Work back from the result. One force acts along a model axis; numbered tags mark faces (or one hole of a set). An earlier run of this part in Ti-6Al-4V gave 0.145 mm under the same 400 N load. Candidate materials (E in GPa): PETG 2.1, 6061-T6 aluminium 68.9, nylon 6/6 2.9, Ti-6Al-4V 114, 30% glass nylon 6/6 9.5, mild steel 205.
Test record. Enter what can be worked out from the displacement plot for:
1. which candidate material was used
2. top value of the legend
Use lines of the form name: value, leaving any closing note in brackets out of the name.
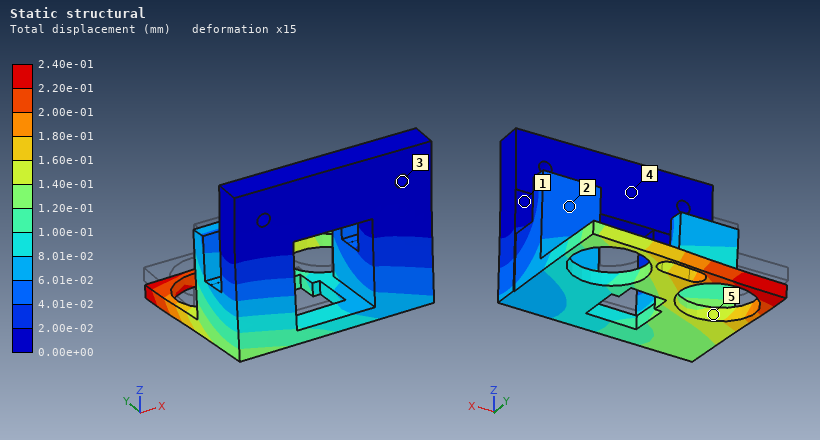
which candidate material was used: 6061-T6 aluminium
top value of the legend: 2.40e-01 mm
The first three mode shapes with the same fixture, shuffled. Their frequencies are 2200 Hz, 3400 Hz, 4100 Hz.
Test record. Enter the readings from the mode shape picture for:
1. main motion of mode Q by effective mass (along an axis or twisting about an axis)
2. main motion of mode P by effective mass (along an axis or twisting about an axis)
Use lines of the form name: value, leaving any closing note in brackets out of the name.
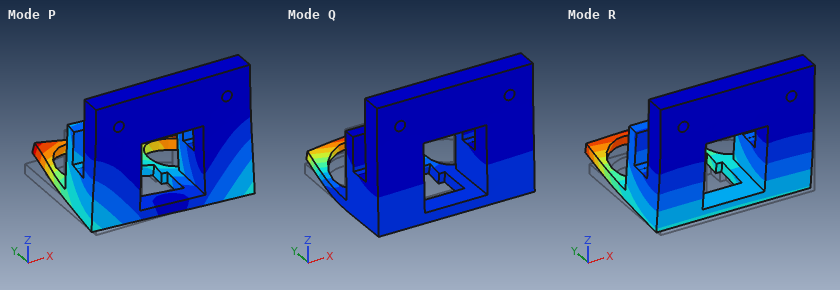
main motion of mode Q by effective mass: along Y
main motion of mode P by effective mass: along X
